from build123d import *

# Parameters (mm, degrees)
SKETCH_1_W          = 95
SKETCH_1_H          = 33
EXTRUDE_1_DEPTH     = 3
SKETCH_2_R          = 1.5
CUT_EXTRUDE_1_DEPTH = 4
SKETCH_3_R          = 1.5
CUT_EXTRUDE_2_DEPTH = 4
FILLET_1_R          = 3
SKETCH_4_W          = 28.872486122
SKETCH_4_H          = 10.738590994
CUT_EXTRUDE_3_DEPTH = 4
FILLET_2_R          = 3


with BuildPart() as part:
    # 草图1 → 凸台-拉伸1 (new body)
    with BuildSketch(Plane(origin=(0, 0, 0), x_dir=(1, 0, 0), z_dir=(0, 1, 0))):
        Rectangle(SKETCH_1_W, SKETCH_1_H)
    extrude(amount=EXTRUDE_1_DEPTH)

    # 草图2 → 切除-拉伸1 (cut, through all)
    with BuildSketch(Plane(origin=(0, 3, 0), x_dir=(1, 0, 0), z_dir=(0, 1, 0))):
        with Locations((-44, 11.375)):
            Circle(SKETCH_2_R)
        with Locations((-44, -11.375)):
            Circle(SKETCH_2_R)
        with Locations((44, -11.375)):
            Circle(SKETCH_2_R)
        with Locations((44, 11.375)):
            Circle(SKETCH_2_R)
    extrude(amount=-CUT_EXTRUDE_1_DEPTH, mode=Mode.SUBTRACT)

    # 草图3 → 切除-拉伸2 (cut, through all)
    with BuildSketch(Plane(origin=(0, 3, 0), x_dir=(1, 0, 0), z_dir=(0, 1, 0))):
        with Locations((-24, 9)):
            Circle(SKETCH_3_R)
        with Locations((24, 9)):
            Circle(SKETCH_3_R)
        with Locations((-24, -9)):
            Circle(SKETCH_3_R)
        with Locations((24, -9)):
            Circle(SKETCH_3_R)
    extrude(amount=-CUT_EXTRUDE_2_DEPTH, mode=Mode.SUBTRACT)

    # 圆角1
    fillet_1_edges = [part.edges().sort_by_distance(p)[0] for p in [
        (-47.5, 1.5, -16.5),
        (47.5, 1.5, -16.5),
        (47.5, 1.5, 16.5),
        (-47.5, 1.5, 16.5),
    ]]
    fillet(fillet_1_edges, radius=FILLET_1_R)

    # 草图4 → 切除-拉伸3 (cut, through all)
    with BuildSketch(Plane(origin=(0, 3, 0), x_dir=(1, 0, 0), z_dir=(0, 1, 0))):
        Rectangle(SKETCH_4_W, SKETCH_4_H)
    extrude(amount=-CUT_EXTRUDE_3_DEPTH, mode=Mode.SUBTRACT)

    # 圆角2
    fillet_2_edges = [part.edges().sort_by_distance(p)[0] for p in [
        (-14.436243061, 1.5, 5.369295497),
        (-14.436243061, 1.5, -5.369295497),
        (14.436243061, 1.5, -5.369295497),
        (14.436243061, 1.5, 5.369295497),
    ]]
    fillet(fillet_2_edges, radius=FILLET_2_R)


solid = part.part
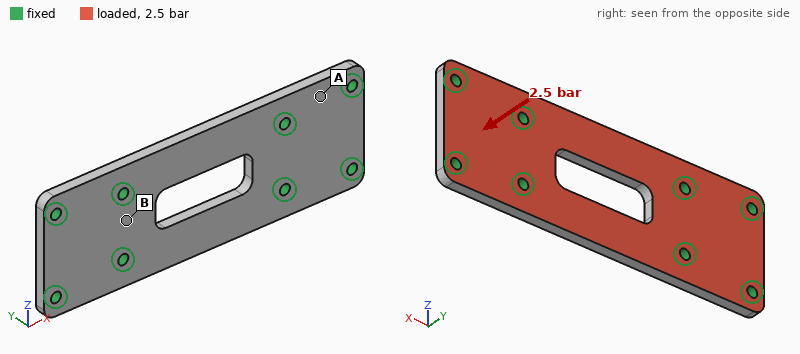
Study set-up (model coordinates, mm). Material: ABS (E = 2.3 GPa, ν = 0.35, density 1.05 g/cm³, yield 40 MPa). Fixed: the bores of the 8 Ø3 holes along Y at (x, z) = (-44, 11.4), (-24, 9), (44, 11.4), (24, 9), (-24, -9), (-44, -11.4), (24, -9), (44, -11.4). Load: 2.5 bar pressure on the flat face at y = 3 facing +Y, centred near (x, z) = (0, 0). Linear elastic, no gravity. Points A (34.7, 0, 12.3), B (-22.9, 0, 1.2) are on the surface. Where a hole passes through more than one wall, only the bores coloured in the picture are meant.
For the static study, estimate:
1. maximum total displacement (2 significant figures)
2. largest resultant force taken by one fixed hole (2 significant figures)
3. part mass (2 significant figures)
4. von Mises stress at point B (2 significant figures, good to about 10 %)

0.63 mm
130 N
8.7 g
9.3 MPa
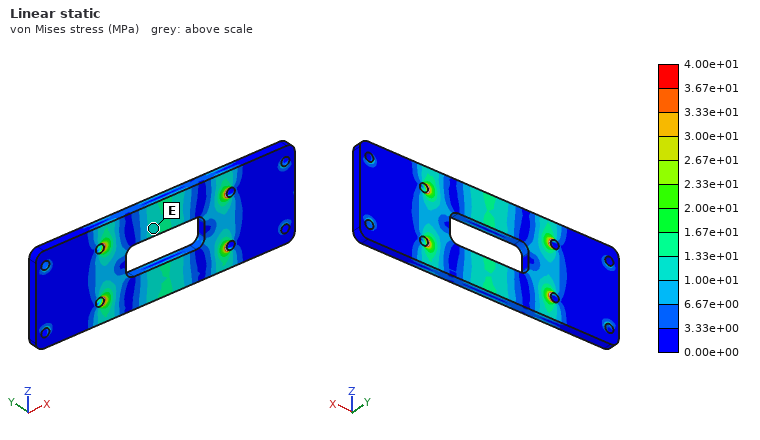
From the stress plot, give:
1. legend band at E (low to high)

1.00e+01 to 1.33e+01 MPa
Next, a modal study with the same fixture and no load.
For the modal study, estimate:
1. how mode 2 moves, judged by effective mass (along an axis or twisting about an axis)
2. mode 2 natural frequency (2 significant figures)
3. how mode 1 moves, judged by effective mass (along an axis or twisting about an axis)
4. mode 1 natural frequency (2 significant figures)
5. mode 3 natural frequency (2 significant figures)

twisting about X
2200 Hz
along Y
2100 Hz
5000 Hz
